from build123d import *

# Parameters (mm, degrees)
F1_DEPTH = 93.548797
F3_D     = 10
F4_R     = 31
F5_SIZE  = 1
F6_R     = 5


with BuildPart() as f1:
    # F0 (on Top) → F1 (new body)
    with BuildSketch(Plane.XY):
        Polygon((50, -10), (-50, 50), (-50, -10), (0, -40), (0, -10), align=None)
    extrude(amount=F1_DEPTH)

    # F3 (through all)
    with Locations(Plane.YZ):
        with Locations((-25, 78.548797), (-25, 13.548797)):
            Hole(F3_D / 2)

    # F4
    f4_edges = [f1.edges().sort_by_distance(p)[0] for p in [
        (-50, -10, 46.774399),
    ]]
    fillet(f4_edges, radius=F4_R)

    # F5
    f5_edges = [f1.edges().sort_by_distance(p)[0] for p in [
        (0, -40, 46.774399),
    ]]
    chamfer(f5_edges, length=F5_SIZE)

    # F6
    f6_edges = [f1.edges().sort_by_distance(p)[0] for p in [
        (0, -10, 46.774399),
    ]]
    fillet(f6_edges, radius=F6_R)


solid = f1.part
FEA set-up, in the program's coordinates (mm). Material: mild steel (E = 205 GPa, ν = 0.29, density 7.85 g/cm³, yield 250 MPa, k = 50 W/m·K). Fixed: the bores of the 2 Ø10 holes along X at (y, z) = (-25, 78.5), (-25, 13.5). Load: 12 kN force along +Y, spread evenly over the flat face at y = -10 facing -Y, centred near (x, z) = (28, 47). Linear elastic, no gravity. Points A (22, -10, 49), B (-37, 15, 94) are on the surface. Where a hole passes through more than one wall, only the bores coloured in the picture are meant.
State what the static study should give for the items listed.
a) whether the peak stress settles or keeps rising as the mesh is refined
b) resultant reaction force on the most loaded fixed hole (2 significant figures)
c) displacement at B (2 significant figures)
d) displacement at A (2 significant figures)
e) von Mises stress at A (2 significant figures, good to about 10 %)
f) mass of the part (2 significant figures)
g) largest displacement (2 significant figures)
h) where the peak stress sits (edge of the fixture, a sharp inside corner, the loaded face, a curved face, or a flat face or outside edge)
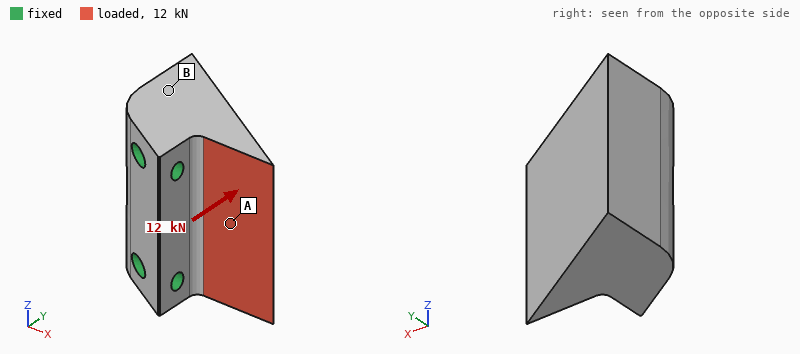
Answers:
keeps rising
6.4 kN
11 µm
17 µm
27 MPa
2.7 kg
47 µm
edge of the fixture
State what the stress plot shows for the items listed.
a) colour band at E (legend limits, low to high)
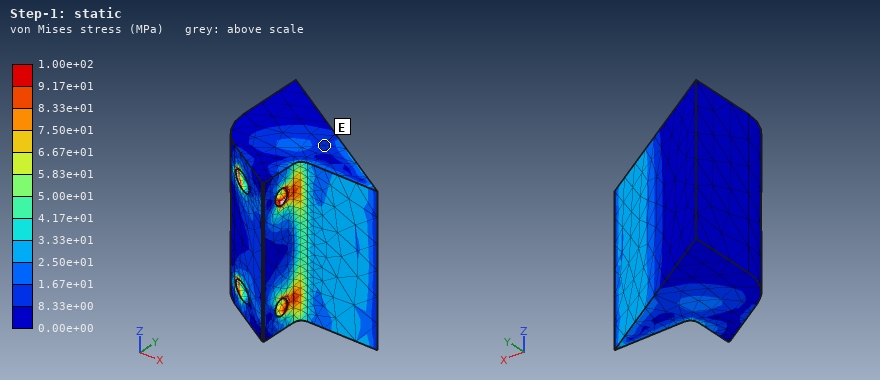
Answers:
8.33e+00 to 1.67e+01 MPa
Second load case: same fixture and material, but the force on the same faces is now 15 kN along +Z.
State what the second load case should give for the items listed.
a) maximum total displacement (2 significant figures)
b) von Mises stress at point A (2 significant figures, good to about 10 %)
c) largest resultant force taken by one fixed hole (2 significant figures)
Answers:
20 µm
22 MPa
11 kN
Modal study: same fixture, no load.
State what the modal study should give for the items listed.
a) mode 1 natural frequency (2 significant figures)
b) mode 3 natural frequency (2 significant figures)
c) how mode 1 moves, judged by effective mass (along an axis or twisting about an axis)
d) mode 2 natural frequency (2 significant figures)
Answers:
3500 Hz
7600 Hz
along X
7300 Hz
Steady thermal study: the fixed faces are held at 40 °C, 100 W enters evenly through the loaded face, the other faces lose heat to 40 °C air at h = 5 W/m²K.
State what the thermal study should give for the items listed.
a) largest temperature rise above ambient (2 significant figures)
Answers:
66 K
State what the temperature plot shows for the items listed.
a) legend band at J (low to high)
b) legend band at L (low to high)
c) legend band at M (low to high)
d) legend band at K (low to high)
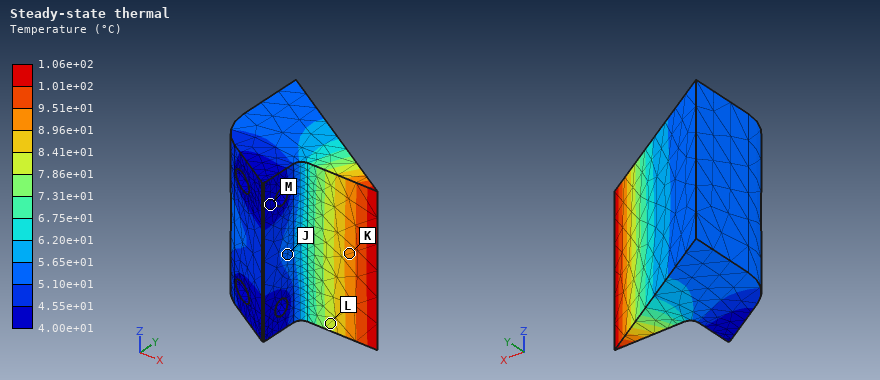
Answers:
5.10e+01 to 5.65e+01 °C
7.86e+01 to 8.41e+01 °C
4.00e+01 to 4.55e+01 °C
8.96e+01 to 9.51e+01 °C
